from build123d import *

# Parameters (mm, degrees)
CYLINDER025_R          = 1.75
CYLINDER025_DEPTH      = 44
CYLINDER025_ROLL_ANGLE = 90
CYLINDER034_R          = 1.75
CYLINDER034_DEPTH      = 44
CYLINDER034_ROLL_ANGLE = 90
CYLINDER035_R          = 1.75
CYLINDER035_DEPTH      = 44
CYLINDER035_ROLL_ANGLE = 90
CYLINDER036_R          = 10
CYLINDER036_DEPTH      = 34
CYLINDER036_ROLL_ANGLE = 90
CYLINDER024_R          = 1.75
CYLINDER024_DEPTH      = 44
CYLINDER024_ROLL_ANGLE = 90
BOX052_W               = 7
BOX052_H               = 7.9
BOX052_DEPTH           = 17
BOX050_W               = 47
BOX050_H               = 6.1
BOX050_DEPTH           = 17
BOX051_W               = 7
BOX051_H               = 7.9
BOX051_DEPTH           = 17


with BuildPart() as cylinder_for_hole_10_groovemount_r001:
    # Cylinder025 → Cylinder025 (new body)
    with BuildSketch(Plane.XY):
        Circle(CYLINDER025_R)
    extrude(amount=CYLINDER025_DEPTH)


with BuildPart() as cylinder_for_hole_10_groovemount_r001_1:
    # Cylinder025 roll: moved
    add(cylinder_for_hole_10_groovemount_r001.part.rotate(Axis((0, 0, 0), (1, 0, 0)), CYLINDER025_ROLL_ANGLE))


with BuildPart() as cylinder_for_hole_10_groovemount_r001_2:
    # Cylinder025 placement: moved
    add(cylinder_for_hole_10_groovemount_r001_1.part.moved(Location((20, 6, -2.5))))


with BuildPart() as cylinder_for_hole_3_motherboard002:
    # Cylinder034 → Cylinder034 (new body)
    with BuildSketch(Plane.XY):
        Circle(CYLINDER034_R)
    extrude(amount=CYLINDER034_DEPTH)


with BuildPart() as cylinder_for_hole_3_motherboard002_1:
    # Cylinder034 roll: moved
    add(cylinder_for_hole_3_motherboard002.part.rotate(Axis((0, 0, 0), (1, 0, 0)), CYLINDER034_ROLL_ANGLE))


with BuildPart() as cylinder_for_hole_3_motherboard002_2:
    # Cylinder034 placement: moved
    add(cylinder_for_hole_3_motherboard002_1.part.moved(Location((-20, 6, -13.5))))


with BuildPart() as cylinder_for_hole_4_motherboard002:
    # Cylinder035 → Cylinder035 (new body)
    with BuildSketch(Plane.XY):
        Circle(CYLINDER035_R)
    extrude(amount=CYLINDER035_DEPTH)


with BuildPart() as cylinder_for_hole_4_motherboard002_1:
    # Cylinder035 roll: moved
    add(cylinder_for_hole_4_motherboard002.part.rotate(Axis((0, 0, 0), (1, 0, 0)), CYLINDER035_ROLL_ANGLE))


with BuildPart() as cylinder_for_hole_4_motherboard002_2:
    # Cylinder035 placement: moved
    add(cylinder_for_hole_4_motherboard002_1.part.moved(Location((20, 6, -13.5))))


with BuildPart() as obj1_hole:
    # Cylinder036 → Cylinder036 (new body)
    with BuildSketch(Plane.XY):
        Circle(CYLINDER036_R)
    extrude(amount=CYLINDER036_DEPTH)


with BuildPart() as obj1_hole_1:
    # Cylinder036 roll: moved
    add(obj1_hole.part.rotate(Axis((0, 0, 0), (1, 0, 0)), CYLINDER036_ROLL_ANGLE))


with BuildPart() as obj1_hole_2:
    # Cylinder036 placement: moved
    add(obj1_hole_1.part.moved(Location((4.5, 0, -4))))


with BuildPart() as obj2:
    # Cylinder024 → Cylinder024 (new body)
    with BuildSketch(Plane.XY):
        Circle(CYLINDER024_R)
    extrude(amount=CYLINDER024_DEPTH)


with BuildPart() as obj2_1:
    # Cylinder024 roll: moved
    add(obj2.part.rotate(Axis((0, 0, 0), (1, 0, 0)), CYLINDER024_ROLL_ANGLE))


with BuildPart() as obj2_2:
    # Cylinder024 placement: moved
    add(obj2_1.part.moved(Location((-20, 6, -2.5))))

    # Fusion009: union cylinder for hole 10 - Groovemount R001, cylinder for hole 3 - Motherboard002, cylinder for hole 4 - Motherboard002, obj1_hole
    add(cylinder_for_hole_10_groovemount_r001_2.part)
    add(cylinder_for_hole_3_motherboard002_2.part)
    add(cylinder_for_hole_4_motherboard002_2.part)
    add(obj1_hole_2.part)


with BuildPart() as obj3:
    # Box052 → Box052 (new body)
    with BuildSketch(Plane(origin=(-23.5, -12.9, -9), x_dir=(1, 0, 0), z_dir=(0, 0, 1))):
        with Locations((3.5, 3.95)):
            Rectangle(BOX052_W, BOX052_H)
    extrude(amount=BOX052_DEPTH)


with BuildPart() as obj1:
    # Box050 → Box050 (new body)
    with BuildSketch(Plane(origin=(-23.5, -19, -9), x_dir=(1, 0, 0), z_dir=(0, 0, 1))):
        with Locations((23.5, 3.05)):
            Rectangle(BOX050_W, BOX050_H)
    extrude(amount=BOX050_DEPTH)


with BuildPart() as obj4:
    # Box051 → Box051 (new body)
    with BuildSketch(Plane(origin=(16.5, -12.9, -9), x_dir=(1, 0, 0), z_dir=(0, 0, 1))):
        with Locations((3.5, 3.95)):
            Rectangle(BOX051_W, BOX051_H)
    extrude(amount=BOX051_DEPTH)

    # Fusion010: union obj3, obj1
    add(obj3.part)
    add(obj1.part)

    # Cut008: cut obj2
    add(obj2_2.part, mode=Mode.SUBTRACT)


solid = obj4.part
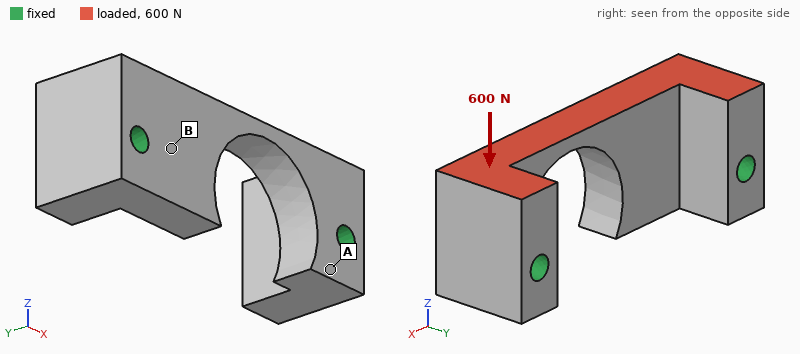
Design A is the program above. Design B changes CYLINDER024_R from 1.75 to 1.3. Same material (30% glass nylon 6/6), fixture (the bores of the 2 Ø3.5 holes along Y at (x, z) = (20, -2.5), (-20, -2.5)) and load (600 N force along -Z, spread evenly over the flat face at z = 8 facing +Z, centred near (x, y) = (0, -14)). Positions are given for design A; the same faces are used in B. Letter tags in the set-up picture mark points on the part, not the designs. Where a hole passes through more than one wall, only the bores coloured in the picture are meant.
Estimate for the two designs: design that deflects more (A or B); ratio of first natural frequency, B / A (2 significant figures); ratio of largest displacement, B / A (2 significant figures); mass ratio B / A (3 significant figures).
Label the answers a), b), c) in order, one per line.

a) B
b) 0.93
c) 1.1
d) 1.01
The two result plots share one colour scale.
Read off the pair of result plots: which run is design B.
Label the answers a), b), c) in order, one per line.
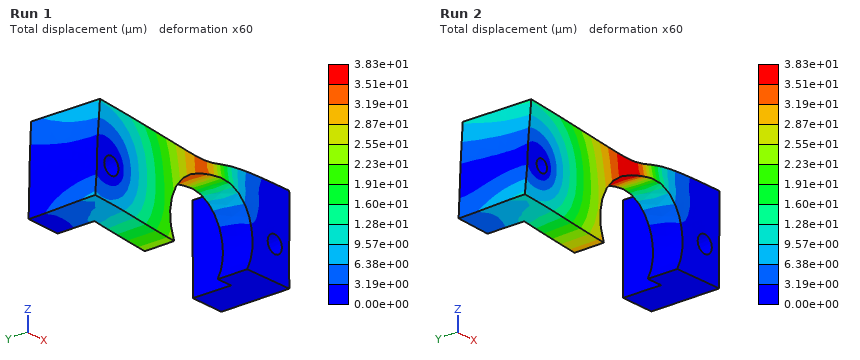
a) Run 2
